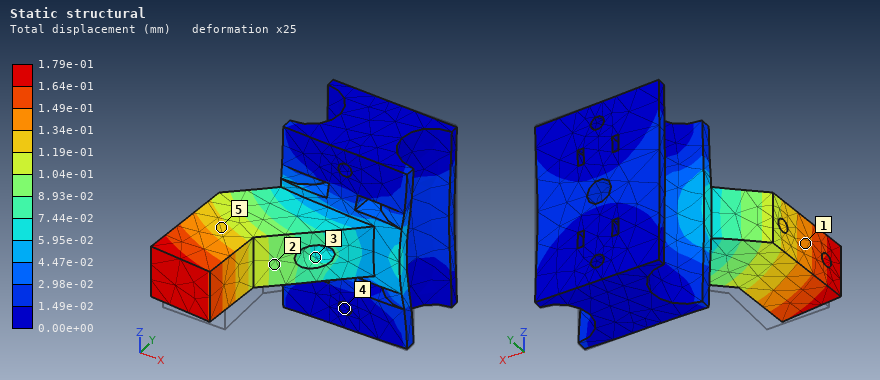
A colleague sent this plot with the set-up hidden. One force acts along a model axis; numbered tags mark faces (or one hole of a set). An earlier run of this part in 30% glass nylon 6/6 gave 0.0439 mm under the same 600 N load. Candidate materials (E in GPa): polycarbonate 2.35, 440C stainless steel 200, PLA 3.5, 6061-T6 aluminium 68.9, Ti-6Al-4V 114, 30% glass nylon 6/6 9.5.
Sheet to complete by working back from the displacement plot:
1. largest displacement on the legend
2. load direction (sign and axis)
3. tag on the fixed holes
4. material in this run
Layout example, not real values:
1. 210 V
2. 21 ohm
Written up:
1. 1.79e-01 mm
2. -X
3. 4
4. polycarbonate
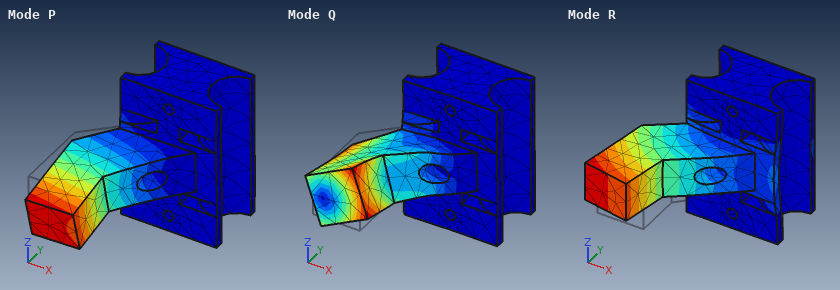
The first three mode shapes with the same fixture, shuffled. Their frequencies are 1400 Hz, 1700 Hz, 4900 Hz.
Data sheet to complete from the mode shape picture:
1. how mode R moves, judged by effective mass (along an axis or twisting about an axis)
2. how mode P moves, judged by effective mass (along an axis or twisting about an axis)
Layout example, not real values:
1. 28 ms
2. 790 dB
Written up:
1. along X
2. along Z
